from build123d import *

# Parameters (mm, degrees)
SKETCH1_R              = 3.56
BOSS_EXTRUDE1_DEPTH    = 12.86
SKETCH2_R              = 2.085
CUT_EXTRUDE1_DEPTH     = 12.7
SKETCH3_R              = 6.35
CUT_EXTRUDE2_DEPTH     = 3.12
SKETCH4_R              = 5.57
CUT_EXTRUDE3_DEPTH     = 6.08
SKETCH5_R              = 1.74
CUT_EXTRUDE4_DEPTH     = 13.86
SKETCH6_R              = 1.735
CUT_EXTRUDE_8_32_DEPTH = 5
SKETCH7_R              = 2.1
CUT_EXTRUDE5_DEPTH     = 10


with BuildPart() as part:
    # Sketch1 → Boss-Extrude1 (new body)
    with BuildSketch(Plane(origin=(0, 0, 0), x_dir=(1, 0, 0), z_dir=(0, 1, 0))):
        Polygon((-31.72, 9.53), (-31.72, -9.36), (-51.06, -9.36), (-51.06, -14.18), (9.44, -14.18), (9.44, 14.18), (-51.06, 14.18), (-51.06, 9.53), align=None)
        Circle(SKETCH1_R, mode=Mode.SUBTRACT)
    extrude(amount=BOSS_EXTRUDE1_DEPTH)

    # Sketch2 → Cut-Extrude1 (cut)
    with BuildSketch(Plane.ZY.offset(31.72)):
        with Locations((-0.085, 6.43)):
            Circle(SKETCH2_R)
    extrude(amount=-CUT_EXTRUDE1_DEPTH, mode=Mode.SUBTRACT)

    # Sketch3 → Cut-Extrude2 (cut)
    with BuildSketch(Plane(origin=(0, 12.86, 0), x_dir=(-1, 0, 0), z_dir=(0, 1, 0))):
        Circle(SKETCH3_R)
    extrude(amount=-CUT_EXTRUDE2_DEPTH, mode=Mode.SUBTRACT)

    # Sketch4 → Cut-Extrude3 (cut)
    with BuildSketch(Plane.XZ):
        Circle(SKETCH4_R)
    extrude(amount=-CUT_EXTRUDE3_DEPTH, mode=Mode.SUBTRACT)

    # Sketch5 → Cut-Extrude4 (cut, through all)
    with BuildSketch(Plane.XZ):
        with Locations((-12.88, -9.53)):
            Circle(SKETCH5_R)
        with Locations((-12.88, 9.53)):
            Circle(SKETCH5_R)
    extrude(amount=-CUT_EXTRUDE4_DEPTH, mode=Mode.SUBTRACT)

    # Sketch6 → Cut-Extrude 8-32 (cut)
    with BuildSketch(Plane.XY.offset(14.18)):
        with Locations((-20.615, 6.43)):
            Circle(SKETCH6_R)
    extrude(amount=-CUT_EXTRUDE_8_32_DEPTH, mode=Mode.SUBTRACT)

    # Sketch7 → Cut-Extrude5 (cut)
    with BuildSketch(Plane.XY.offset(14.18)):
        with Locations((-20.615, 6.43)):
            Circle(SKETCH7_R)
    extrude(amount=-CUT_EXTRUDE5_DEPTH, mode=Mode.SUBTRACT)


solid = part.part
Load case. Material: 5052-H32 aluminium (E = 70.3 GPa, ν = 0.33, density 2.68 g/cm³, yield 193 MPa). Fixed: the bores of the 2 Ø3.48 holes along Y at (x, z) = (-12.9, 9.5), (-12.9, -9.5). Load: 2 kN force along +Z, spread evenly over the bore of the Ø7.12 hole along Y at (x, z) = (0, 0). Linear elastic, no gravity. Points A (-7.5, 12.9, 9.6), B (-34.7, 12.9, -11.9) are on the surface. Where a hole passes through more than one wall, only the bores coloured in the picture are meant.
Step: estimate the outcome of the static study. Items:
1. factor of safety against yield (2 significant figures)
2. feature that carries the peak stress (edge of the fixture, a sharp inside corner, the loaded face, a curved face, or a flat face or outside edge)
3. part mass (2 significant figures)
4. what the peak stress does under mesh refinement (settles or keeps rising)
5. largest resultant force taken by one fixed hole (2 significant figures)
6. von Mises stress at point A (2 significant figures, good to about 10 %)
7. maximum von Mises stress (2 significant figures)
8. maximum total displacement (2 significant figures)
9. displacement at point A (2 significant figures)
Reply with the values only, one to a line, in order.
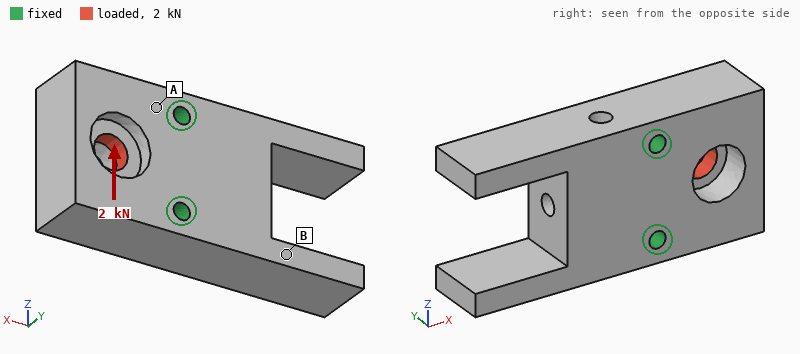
3.6
the loaded face
42 g
settles
1.5 kN
10 MPa
53 MPa
9.9 µm
1.8 µm
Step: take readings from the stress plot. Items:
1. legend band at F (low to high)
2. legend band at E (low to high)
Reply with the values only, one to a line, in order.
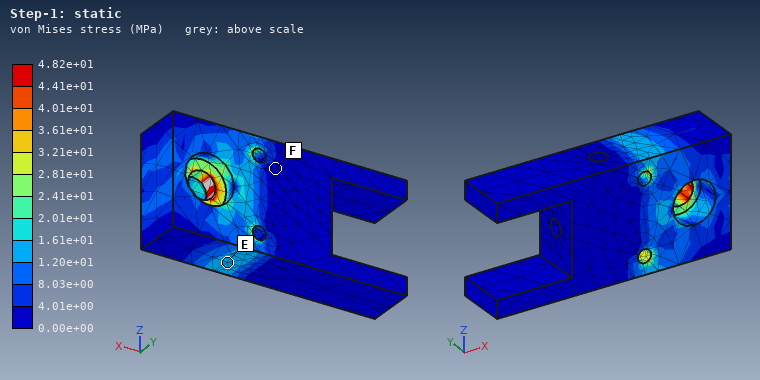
0.00e+00 to 4.01e+00 MPa
1.20e+01 to 1.61e+01 MPa
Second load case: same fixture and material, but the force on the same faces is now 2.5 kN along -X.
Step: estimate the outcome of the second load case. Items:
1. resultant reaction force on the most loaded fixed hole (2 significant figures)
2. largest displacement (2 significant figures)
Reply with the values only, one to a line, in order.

1.3 kN
6.5 µm
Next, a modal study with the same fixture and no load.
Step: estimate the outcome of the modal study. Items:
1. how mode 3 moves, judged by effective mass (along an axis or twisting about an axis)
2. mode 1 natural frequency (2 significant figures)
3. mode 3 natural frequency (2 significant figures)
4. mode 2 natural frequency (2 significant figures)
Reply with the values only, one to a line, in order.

along Y
7500 Hz
9200 Hz
7800 Hz
